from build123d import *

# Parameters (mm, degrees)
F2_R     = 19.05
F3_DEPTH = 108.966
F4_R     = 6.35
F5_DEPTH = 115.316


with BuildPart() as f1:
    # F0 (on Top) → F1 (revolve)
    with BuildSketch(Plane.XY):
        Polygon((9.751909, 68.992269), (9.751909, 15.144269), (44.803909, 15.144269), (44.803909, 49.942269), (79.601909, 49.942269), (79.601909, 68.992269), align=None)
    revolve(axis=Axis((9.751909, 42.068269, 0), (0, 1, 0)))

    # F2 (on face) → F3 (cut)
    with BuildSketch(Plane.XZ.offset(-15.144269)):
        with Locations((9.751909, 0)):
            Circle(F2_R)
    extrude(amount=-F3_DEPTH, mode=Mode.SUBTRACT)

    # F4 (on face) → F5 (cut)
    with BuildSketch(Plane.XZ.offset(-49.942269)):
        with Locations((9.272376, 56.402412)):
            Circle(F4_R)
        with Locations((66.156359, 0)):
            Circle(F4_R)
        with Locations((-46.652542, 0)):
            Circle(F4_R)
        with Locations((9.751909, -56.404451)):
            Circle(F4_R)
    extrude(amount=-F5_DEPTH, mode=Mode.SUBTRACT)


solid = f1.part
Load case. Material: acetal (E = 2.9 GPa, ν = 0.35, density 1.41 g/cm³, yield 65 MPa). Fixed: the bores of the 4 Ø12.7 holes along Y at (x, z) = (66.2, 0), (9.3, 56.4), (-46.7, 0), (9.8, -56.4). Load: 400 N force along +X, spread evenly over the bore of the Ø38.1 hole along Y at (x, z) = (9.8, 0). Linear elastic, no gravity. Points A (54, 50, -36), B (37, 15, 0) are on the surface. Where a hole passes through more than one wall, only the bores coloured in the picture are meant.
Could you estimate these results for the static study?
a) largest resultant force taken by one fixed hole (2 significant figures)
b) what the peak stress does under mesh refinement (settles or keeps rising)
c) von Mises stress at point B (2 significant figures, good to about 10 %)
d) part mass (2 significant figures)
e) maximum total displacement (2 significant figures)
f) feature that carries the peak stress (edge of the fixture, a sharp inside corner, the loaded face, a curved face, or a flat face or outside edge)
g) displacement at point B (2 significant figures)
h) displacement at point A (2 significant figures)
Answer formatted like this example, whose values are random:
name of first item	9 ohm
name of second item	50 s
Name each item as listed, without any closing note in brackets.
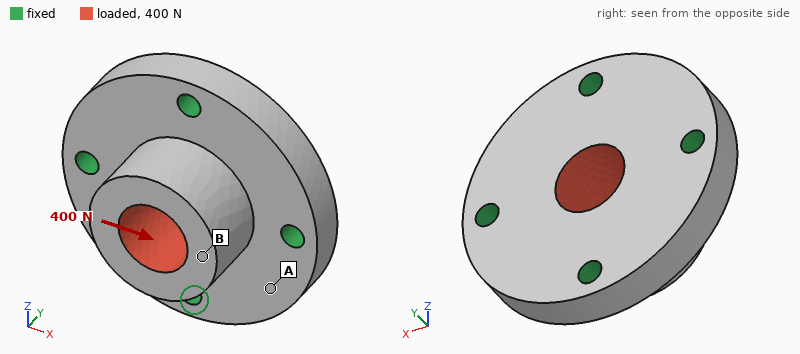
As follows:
largest resultant force taken by one fixed hole	140 N
what the peak stress does under mesh refinement	keeps rising
von Mises stress at point B	0.13 MPa
part mass	500 g
maximum total displacement	9.1 µm
feature that carries the peak stress	edge of the fixture
displacement at point B	8.8 µm
displacement at point A	2.0 µm
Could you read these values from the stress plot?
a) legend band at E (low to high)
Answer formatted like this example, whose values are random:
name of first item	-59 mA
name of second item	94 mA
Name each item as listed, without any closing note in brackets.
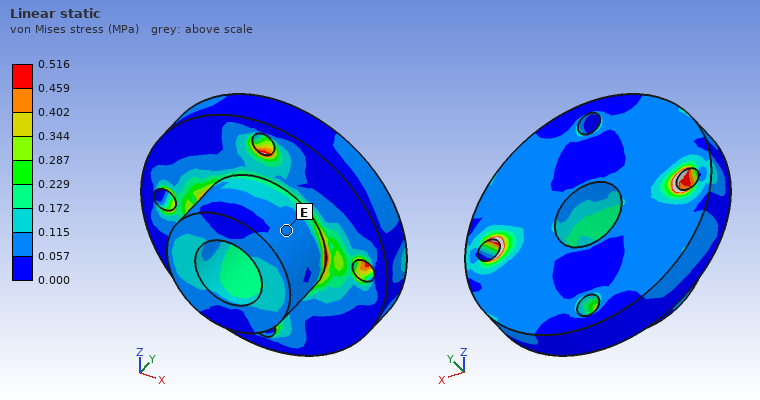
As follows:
legend band at E	0.057 to 0.115 MPa
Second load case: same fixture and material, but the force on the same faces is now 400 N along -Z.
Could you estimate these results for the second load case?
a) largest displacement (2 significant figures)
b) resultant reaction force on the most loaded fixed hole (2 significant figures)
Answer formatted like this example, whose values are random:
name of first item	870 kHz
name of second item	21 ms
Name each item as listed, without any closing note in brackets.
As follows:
largest displacement	9.1 µm
resultant reaction force on the most loaded fixed hole	140 N
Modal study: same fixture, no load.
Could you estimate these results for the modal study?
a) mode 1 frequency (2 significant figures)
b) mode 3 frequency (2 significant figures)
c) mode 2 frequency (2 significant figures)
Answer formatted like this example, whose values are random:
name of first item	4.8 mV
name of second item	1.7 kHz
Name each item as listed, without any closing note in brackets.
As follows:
mode 1 frequency	2400 Hz
mode 3 frequency	2500 Hz
mode 2 frequency	2500 Hz
